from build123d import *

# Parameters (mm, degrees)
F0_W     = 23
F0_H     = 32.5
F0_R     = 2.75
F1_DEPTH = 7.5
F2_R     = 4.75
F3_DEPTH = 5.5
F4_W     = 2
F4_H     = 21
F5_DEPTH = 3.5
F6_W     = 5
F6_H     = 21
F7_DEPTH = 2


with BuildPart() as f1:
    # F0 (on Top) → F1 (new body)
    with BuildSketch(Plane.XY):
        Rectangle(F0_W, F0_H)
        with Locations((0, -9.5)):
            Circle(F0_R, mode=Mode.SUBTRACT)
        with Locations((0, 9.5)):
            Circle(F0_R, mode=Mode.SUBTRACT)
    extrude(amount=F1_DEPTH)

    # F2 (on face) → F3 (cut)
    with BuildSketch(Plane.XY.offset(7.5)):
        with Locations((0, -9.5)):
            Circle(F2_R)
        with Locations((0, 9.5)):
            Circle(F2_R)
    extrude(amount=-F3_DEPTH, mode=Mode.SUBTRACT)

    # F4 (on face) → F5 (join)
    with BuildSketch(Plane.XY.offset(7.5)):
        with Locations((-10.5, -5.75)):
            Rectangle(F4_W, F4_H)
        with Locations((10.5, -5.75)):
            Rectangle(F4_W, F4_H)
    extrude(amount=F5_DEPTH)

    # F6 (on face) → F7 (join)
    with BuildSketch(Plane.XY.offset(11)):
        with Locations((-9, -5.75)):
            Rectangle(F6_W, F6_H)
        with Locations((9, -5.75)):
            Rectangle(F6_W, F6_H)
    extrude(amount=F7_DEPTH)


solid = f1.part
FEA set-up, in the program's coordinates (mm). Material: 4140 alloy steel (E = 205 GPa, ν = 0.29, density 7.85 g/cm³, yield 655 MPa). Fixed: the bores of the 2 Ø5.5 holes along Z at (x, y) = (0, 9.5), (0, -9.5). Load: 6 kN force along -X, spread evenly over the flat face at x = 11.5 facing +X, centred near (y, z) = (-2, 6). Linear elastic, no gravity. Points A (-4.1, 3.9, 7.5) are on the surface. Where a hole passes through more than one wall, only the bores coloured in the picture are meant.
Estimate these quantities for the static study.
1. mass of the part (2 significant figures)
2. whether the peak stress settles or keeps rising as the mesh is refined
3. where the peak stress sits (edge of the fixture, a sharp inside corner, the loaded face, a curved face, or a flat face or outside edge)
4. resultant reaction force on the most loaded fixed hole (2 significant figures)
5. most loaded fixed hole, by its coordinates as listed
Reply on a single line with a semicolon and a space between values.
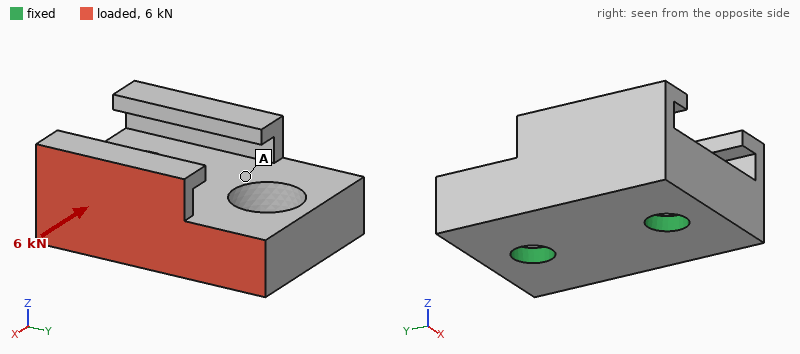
43 g; keeps rising; edge of the fixture; 3.4 kN; (0, -9.5)
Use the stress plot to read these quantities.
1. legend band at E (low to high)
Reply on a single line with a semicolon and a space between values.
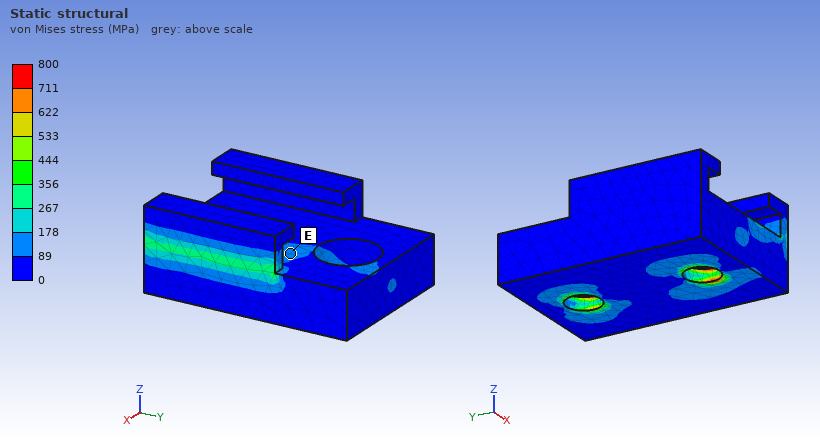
89 to 178 MPa
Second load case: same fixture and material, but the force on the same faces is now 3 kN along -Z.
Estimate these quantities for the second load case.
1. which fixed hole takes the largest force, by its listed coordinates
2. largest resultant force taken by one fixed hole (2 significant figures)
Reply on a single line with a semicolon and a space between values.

(0, -9.5); 1.8 kN
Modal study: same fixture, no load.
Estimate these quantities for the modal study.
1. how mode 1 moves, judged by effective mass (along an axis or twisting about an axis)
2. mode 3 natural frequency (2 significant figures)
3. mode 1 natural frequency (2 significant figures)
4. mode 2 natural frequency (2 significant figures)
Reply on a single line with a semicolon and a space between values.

along X; 21 kHz; 8900 Hz; 20 kHz
